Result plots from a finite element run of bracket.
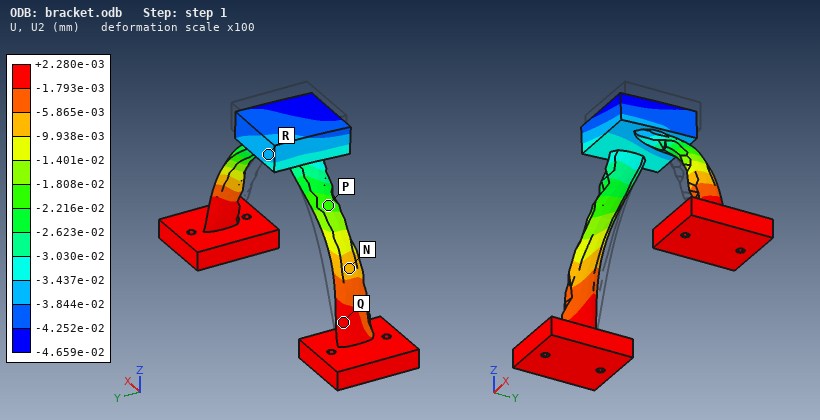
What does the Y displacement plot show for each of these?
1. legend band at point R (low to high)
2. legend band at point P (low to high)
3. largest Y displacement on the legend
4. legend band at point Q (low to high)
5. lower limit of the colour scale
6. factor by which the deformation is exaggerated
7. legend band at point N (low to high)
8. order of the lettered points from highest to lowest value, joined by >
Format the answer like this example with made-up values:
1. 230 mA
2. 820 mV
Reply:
1. -3.844e-02 to -3.437e-02 mm
2. -2.216e-02 to -1.808e-02 mm
3. +2.280e-03 mm
4. -1.793e-03 to +2.280e-03 mm
5. -4.659e-02 mm
6. 100
7. -9.938e-03 to -5.865e-03 mm
8. Q > N > P > R
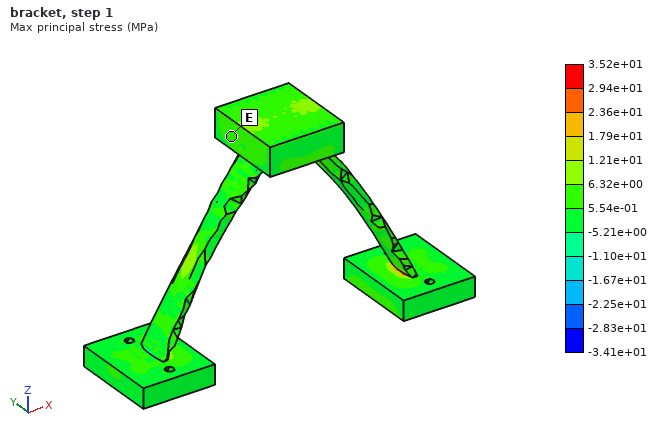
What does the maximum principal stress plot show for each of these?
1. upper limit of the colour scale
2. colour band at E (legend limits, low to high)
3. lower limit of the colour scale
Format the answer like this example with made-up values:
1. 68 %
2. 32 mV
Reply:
1. 3.52e+01 MPa
2. 5.54e-01 to 6.32e+00 MPa
3. -3.41e+01 MPa
